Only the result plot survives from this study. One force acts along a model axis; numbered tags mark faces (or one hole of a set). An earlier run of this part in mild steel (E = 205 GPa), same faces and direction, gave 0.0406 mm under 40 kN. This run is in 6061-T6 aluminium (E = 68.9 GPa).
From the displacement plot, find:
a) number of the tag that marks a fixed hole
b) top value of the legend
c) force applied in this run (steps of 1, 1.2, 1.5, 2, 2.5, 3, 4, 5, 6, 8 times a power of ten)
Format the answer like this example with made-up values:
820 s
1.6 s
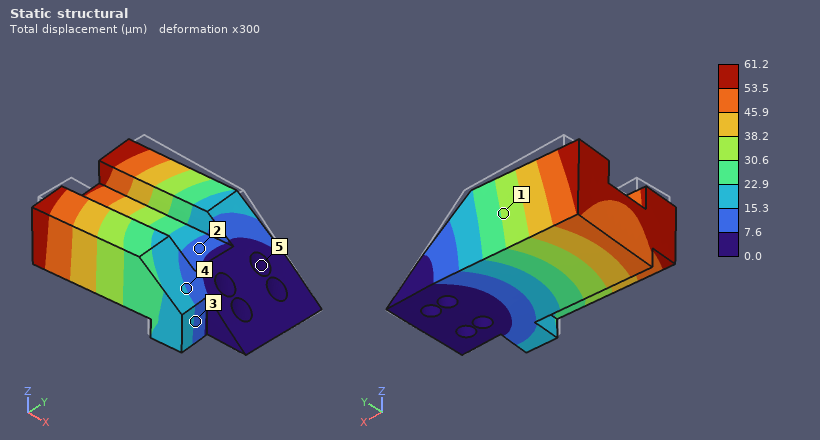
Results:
5
61.2 µm
20 kN
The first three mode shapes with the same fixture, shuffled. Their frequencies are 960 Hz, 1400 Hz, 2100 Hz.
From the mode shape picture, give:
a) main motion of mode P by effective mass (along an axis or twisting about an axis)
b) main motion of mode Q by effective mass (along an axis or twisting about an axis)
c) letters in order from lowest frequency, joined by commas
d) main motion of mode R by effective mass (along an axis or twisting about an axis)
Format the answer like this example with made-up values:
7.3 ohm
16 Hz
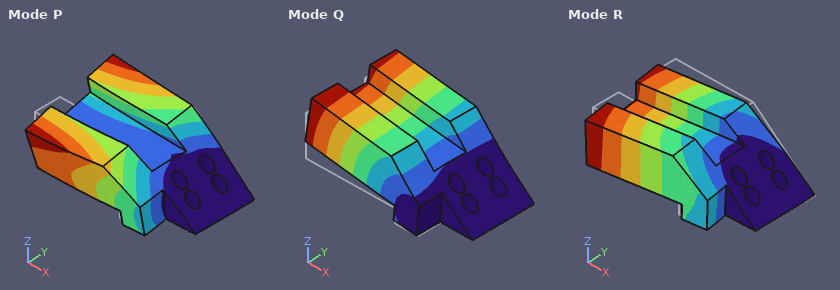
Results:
twisting about X
along Z
Q, R, P
along Y
